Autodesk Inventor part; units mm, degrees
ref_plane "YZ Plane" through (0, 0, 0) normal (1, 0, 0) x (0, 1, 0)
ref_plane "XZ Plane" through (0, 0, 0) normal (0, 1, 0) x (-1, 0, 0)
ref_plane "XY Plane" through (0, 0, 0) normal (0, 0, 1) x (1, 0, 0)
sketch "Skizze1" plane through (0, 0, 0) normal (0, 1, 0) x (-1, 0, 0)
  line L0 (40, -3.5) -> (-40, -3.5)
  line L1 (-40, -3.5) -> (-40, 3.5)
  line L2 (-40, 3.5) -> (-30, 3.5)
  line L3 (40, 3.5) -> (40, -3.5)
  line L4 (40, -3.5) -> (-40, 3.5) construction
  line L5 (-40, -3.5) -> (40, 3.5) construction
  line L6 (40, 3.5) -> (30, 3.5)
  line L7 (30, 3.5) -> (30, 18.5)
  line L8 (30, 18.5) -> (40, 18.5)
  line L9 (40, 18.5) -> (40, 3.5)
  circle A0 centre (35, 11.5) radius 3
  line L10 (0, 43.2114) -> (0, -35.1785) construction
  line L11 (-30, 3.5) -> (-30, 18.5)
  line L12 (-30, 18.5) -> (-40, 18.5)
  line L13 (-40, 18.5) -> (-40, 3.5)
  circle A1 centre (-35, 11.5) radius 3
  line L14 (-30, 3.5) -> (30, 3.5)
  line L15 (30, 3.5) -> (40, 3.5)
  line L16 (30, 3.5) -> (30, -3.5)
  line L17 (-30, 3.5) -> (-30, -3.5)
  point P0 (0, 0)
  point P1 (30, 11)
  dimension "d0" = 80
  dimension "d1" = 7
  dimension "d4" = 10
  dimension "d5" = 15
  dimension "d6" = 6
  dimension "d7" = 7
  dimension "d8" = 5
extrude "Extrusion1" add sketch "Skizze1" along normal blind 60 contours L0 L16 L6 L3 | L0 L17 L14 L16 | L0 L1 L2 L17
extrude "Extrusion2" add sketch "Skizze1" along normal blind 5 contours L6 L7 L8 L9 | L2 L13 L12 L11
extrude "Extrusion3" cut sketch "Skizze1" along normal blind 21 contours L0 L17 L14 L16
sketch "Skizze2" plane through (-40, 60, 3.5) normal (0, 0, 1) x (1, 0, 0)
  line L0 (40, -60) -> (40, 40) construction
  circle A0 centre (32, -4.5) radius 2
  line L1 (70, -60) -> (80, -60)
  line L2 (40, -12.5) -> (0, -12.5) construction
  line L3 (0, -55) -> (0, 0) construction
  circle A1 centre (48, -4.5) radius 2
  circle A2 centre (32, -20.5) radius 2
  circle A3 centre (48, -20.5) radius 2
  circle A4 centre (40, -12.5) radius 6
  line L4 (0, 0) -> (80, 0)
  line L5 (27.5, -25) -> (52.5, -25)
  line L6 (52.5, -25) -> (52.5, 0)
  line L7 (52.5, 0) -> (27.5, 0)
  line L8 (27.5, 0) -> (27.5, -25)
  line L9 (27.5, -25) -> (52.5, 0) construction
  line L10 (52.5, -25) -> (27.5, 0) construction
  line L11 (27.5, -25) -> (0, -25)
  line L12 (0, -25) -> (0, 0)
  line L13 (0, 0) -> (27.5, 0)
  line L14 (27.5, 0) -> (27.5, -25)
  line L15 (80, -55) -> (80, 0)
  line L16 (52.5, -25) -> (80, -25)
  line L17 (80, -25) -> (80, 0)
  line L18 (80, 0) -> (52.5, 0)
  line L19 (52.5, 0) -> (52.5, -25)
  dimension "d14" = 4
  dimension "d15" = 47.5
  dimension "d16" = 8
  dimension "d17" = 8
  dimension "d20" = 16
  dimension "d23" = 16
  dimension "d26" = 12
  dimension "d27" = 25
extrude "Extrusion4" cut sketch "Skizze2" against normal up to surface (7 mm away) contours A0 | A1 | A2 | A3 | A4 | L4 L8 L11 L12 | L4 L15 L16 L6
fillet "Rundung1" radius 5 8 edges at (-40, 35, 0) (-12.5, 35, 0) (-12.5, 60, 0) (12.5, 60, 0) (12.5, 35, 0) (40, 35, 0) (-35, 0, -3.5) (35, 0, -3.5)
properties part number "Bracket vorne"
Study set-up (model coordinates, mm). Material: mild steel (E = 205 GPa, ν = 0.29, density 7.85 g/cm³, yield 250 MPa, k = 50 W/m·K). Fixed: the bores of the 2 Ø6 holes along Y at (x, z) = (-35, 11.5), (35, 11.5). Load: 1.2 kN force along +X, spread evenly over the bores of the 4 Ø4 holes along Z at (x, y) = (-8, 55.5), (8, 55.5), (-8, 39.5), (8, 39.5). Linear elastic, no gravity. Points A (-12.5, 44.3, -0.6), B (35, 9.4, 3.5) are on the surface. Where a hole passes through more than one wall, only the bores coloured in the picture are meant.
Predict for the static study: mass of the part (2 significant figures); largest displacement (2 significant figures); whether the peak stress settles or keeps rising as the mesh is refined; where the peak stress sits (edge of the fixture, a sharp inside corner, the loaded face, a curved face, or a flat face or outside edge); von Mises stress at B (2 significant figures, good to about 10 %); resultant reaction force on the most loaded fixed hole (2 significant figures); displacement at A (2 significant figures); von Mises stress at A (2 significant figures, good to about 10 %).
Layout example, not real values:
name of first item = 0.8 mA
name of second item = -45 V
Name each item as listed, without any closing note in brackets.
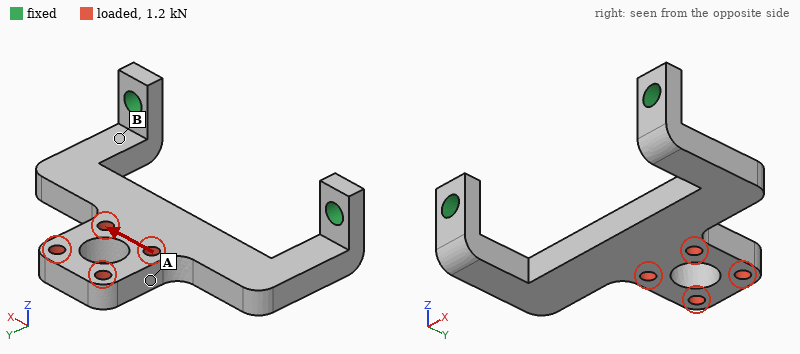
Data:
mass of the part = 120 g
largest displacement = 41 µm
whether the peak stress settles or keeps rising as the mesh is refined = keeps rising
where the peak stress sits = edge of the fixture
von Mises stress at B = 53 MPa
resultant reaction force on the most loaded fixed hole = 900 N
displacement at A = 32 µm
von Mises stress at A = 21 MPa
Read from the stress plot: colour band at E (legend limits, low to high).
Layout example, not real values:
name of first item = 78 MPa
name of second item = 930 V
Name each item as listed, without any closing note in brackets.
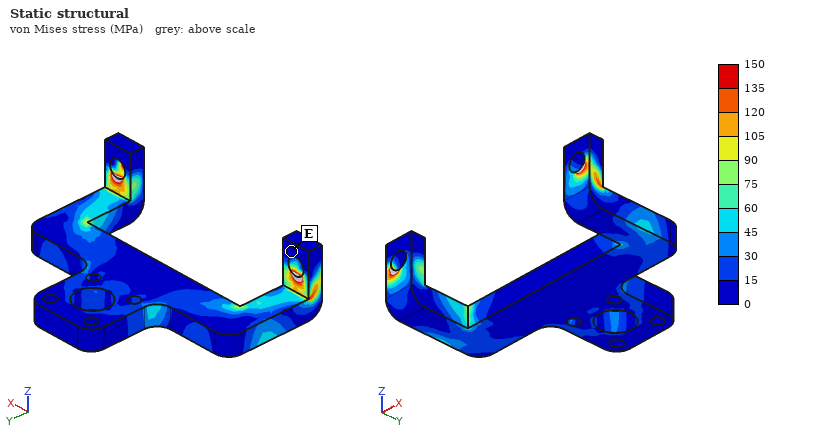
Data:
colour band at E = 0 to 15 MPa
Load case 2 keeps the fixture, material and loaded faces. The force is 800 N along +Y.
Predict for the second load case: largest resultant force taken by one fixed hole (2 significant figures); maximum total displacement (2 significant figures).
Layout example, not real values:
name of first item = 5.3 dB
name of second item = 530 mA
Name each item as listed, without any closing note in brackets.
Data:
largest resultant force taken by one fixed hole = 430 N
maximum total displacement = 52 µm
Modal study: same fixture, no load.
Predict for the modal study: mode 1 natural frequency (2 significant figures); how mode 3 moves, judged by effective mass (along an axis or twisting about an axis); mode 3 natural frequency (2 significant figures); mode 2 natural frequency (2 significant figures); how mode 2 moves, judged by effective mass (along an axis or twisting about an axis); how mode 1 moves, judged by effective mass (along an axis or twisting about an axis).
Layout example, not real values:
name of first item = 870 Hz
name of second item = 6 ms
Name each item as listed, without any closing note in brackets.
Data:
mode 1 natural frequency = 930 Hz
how mode 3 moves, judged by effective mass = along X
mode 3 natural frequency = 3800 Hz
mode 2 natural frequency = 3200 Hz
how mode 2 moves, judged by effective mass = along X
how mode 1 moves, judged by effective mass = along Z
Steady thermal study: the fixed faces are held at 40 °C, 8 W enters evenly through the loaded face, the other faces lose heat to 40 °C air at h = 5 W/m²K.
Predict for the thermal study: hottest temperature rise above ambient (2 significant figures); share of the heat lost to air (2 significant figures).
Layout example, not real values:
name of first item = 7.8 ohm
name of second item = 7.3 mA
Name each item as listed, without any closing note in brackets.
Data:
hottest temperature rise above ambient = 69 K
share of the heat lost to air = 16 %
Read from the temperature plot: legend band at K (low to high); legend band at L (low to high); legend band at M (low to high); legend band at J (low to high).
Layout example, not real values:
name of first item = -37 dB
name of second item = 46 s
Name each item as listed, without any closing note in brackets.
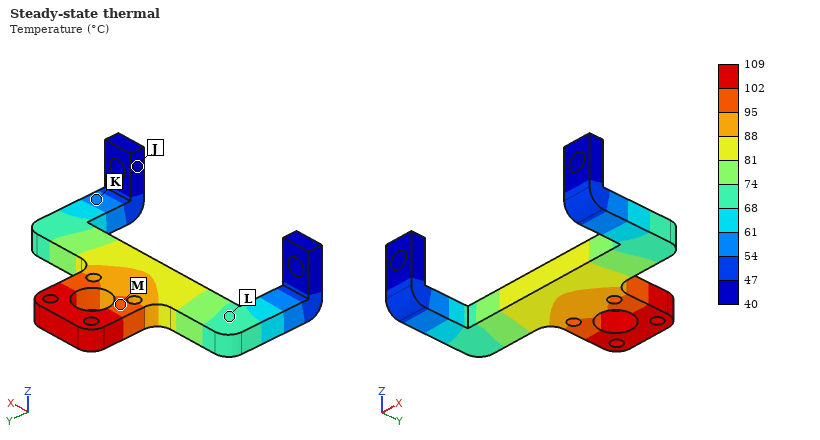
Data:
legend band at K = 54 to 61 °C
legend band at L = 68 to 74 °C
legend band at M = 95 to 102 °C
legend band at J = 40 to 47 °C
